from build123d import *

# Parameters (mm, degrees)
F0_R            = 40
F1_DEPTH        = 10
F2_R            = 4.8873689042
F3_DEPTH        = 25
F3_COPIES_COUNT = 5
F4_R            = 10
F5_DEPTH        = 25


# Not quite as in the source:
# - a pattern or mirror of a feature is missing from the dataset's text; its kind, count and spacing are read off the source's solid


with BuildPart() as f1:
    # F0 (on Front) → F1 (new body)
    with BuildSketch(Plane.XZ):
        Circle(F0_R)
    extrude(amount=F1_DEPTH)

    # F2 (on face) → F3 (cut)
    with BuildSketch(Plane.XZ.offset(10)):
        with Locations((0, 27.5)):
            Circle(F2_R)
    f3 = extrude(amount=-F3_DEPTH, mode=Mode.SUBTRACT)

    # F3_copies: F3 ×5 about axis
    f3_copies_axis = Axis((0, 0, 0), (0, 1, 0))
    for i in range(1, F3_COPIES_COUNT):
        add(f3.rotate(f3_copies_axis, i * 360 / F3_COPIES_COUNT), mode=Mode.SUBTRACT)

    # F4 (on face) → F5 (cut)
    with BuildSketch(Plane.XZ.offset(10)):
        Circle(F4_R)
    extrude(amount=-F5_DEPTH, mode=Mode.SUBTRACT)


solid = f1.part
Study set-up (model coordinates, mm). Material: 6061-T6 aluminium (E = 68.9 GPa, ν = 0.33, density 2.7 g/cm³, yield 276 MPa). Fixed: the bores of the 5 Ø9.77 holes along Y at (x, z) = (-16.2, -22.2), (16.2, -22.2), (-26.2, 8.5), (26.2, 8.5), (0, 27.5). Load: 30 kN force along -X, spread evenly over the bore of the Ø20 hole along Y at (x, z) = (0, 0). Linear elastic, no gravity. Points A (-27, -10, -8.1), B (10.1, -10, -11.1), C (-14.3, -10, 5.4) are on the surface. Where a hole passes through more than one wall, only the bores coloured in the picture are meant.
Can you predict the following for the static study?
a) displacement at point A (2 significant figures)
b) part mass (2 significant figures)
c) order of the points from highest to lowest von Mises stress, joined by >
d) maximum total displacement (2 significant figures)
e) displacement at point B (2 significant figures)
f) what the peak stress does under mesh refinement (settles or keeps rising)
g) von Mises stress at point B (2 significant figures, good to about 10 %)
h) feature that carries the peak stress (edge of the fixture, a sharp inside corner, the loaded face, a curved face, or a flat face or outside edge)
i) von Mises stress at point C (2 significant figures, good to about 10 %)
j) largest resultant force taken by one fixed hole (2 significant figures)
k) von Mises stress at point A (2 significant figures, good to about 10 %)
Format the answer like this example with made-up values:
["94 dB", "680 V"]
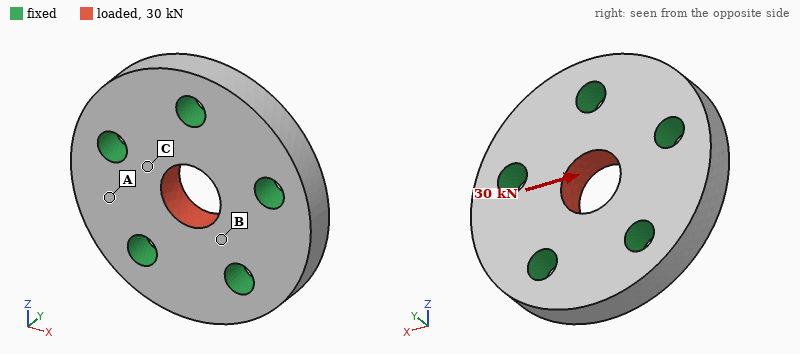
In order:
["4.6 µm", "120 g", "C > B > A", "12 µm", "6.6 µm", "keeps rising", "36 MPa", "edge of the fixture", "54 MPa", "8.5 kN", "13 MPa"]
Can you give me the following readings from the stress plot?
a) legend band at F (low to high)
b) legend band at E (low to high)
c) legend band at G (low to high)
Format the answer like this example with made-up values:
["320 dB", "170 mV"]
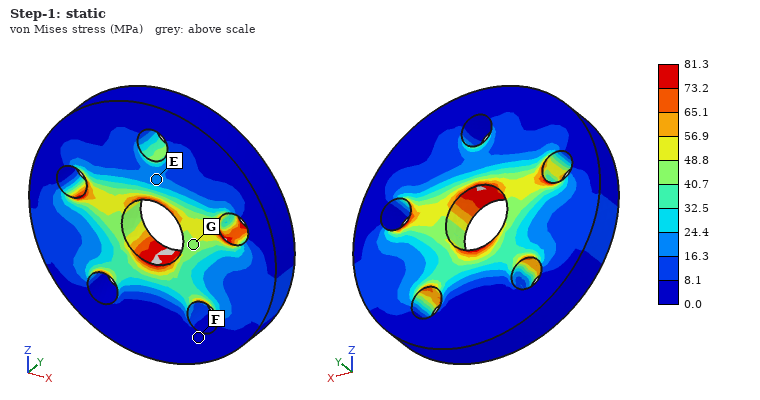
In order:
["0.0 to 8.1 MPa", "16.3 to 24.4 MPa", "40.7 to 48.8 MPa"]
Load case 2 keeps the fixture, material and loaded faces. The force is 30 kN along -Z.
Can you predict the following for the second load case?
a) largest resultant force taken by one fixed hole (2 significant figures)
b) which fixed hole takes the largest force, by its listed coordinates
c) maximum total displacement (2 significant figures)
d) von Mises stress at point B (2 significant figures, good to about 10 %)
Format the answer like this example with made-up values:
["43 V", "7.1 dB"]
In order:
["8.8 kN", "(0, 27.5)", "12 µm", "47 MPa"]
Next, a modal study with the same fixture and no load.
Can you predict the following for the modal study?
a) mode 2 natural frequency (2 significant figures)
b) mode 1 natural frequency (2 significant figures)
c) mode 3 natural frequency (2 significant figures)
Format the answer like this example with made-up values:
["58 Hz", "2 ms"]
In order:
["27 kHz", "27 kHz", "28 kHz"]
